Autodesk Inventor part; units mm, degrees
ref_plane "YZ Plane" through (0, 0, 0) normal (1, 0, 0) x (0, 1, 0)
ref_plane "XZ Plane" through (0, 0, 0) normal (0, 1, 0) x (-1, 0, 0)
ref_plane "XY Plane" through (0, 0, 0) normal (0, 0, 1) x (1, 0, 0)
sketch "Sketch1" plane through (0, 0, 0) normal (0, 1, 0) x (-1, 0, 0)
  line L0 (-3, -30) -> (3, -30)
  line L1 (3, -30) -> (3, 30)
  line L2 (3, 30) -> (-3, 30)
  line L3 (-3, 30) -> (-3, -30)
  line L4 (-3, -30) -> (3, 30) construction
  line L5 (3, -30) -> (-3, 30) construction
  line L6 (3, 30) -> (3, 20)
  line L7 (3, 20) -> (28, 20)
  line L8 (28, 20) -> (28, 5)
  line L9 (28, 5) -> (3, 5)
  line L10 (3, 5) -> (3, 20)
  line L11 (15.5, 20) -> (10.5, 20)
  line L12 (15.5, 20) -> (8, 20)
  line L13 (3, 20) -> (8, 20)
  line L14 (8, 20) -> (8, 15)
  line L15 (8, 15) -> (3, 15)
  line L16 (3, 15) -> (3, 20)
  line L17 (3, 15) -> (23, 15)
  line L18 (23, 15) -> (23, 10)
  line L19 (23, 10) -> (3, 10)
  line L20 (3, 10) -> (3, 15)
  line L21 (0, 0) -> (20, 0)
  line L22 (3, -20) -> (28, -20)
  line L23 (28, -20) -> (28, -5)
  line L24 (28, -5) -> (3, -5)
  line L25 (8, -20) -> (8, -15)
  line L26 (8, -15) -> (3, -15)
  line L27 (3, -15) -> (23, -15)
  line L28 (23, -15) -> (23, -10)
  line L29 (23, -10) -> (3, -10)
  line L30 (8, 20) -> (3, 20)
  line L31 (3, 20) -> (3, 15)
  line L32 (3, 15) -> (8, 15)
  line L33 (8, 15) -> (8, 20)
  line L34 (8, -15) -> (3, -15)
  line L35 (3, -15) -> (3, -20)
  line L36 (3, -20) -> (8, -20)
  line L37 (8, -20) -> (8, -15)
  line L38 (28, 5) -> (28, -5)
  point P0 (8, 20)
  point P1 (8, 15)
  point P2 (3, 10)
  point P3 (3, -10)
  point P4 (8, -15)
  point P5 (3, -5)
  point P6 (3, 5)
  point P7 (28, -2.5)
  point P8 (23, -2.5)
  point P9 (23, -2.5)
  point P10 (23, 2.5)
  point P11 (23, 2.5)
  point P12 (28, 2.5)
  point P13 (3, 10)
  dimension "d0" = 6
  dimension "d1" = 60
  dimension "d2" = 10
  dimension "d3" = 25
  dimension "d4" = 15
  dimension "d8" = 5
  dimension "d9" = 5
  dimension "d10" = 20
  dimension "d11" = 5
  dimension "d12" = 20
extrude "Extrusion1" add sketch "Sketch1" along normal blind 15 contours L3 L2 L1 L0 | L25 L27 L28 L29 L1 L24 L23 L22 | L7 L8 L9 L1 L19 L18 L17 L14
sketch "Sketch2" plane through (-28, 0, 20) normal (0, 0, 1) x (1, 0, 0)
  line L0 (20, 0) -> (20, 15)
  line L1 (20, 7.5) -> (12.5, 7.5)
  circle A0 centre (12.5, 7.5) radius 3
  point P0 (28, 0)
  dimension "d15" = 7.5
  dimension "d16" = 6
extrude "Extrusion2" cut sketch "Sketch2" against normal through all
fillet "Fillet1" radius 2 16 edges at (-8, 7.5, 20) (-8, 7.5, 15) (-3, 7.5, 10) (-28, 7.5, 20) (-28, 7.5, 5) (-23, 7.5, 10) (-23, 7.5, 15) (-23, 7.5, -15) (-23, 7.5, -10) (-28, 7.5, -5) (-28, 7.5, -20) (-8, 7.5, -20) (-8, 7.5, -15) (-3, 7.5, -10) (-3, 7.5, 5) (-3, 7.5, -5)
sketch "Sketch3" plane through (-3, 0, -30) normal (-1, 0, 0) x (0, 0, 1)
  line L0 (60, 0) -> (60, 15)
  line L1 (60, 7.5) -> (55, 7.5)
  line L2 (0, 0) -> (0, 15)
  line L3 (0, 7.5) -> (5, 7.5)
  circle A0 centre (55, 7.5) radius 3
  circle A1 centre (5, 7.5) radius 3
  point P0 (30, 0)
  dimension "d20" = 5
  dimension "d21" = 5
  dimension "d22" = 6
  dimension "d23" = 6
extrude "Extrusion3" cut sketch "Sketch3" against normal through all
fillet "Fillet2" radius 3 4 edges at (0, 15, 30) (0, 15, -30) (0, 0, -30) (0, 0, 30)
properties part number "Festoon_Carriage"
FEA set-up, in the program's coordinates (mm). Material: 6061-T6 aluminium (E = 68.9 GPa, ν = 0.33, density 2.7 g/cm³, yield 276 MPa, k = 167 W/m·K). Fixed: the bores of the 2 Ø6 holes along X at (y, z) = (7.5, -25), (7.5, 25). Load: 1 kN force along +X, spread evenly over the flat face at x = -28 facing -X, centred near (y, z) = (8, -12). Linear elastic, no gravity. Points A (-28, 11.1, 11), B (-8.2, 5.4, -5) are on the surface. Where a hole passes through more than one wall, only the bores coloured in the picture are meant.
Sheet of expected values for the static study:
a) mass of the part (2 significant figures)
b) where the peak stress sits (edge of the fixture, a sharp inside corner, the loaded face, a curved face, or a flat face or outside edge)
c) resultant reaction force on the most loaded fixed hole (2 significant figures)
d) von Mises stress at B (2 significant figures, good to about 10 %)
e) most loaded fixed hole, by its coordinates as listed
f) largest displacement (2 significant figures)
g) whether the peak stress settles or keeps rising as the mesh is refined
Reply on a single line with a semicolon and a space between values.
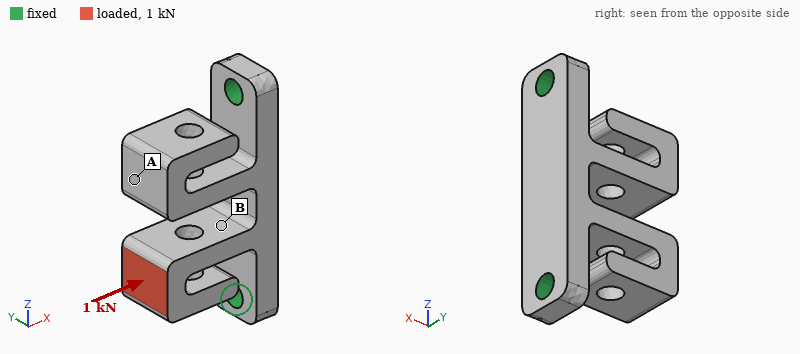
32 g; a sharp inside corner; 860 N; 61 MPa; (7.5, -25); 0.24 mm; keeps rising
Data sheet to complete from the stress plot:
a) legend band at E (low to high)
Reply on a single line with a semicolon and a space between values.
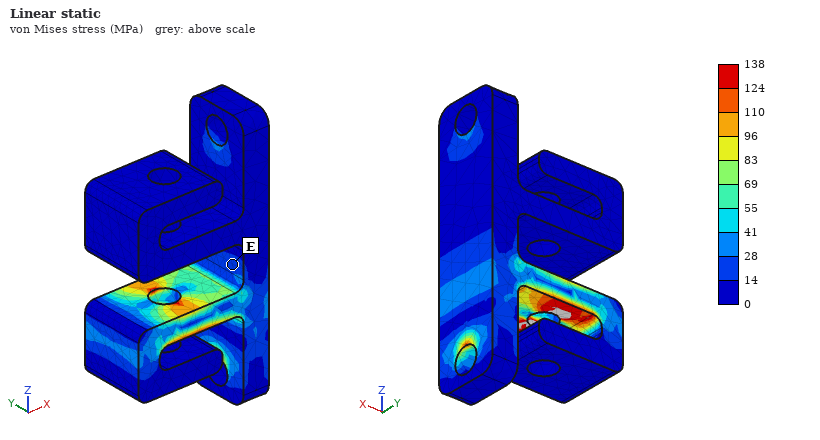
14 to 28 MPa
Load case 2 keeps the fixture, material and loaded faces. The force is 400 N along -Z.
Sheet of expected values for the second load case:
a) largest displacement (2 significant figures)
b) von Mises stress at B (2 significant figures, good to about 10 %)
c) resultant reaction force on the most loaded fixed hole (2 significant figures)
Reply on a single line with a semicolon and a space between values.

0.32 mm; 110 MPa; 380 N
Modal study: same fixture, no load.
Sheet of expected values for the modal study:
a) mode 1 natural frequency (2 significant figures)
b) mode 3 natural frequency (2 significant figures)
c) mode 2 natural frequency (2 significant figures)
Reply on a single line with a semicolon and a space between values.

2800 Hz; 3000 Hz; 2900 Hz
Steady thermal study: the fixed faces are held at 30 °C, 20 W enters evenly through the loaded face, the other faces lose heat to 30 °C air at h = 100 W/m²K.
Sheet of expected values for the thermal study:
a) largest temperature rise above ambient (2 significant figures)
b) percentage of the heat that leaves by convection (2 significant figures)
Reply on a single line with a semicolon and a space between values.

44 K; 38 %
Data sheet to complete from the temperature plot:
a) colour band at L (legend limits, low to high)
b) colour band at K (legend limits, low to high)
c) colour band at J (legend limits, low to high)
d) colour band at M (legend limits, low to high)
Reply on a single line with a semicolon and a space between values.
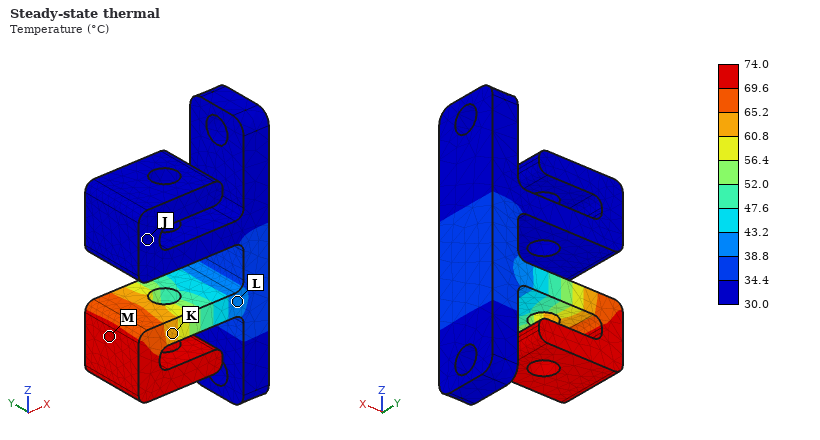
38.8 to 43.2 °C; 60.8 to 65.2 °C; 30.0 to 34.4 °C; 69.6 to 74.0 °C
